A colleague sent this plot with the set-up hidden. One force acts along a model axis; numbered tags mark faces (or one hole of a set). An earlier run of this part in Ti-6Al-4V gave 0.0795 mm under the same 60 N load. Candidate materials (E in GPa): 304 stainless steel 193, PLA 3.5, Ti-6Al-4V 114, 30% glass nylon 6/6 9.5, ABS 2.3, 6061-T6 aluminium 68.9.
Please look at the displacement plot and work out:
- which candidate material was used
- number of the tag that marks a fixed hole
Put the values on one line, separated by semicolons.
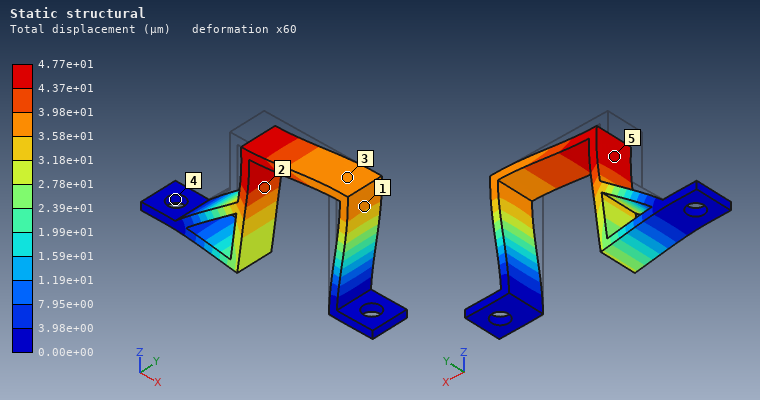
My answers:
304 stainless steel; 4
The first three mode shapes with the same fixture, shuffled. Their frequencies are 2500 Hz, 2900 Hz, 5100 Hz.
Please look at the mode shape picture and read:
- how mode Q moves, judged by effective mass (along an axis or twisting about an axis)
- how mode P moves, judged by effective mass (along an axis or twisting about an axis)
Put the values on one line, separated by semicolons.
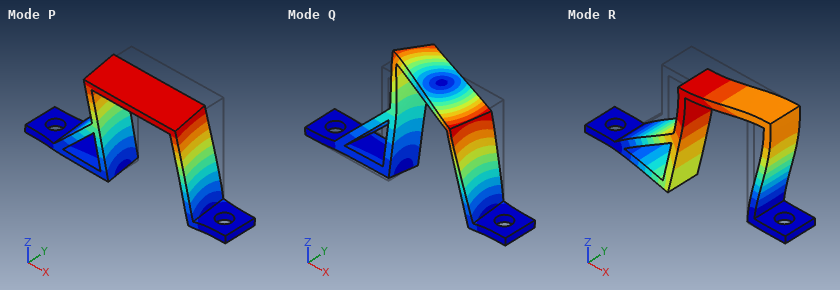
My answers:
twisting about Z; along Y
